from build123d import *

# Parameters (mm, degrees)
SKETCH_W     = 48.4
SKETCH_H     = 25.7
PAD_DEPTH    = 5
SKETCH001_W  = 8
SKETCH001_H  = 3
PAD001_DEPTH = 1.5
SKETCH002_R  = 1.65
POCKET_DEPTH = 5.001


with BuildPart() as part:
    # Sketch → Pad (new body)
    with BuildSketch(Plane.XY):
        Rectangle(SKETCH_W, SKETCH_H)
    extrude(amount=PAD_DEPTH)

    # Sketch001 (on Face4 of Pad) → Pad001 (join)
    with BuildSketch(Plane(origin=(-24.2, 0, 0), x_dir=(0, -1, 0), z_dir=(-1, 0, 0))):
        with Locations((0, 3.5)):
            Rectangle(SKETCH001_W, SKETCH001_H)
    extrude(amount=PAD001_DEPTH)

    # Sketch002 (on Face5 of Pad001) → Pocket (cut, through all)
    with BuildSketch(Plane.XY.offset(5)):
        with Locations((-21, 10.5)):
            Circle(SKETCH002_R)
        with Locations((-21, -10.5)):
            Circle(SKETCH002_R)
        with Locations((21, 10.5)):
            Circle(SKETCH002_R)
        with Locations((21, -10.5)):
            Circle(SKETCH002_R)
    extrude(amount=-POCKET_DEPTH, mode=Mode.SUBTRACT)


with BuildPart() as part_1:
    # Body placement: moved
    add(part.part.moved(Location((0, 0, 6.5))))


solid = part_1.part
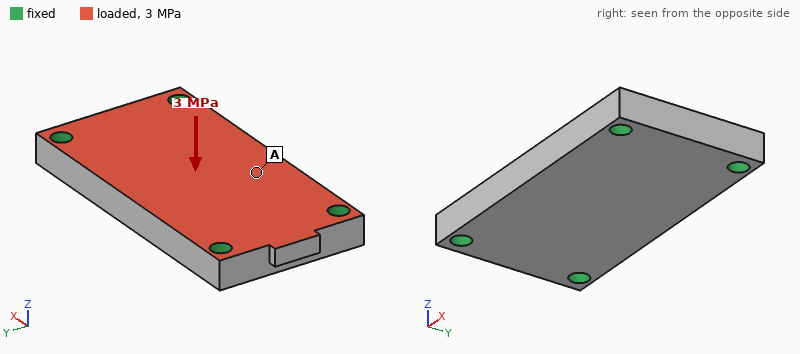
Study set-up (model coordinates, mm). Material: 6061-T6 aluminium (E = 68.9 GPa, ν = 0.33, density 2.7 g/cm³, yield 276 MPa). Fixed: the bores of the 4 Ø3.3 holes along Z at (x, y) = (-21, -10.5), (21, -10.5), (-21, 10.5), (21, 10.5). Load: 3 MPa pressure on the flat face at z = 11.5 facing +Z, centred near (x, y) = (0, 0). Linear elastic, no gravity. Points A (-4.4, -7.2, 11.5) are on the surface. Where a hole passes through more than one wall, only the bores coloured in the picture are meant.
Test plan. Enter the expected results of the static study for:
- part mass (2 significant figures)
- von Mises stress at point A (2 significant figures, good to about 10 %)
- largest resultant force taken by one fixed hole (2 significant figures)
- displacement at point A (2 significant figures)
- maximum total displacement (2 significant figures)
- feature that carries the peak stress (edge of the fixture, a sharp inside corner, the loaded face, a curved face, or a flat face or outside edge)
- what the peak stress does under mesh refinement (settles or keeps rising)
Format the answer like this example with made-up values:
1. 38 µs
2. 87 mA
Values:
1. 16 g
2. 46 MPa
3. 930 N
4. 41 µm
5. 46 µm
6. edge of the fixture
7. keeps rising
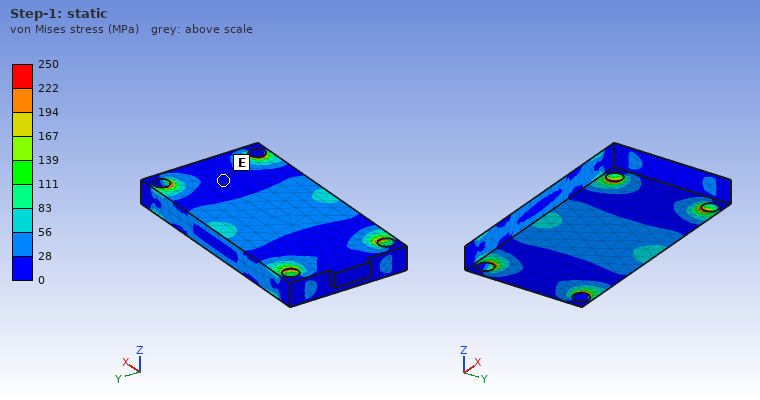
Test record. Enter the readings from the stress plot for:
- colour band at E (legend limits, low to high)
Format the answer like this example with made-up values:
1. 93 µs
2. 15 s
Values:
1. 0 to 28 MPa
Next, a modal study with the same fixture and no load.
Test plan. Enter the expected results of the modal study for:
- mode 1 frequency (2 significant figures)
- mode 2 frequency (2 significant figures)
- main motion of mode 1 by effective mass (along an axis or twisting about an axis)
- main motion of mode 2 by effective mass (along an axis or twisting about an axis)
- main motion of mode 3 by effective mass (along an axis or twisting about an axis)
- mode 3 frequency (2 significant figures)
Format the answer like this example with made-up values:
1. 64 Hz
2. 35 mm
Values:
1. 13 kHz
2. 20 kHz
3. along Z
4. twisting about X
5. along Y
6. 31 kHz
